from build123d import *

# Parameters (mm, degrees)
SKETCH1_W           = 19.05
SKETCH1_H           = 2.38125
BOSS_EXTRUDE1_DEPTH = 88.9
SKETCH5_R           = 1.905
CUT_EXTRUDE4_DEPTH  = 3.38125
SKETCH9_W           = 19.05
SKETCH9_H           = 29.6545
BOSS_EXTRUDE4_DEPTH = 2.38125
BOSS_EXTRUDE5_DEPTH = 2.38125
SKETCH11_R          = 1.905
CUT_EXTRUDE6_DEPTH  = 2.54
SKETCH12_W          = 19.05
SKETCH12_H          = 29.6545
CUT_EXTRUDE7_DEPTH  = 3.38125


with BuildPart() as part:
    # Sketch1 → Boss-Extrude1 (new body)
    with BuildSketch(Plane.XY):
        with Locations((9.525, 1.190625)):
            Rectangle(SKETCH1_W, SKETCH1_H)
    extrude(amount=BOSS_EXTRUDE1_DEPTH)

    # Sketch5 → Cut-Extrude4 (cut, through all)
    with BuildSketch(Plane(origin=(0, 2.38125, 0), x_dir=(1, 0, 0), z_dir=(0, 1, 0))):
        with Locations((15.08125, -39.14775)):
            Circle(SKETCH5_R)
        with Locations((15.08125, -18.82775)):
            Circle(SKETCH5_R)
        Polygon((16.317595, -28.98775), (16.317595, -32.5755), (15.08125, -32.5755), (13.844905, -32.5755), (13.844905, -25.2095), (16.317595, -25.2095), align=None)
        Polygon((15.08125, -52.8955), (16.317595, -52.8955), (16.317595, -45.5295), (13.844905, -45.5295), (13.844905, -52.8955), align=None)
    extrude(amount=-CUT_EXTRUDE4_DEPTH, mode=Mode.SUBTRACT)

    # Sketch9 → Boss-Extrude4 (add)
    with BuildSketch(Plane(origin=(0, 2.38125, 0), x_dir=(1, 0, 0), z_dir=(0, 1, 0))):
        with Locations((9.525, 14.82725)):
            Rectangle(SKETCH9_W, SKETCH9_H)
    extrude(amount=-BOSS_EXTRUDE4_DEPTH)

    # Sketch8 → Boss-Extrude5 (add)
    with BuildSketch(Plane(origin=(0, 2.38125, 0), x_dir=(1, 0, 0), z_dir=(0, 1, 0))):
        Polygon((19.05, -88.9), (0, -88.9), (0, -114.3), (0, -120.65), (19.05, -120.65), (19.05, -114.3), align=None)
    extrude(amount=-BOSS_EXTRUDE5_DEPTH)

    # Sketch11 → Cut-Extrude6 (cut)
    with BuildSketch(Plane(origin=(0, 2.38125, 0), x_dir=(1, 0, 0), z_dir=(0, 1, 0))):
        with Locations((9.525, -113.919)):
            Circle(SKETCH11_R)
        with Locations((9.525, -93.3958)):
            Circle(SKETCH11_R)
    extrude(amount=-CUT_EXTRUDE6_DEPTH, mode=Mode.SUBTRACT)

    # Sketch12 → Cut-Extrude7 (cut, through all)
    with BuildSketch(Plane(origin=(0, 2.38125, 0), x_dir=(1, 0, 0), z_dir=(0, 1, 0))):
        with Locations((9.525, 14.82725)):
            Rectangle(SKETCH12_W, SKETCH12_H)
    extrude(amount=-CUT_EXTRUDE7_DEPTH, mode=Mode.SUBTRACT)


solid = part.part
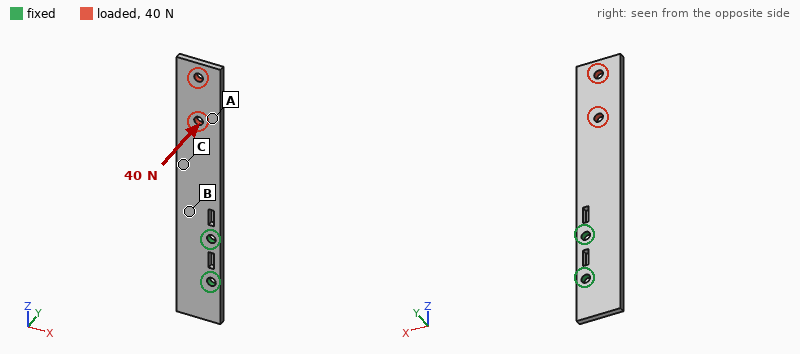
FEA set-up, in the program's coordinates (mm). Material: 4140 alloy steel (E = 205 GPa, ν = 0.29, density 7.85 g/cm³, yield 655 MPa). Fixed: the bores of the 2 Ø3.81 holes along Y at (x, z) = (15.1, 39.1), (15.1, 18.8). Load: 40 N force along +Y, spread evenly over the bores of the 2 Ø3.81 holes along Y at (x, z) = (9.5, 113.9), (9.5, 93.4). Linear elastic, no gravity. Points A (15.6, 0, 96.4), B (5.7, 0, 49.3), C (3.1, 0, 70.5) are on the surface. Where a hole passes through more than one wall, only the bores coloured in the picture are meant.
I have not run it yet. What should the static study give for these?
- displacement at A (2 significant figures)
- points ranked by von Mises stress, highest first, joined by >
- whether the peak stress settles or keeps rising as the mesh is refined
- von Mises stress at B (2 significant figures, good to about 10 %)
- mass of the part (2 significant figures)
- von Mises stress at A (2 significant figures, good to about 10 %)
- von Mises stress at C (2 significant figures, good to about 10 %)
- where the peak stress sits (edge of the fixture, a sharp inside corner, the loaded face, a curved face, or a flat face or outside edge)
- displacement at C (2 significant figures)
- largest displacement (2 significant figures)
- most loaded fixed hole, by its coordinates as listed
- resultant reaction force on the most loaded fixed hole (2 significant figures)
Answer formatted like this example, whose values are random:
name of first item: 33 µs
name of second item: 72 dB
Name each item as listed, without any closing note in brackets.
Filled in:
displacement at A: 0.73 mm
points ranked by von Mises stress, highest first, joined by >: B > C > A
whether the peak stress settles or keeps rising as the mesh is refined: keeps rising
von Mises stress at B: 130 MPa
mass of the part: 41 g
von Mises stress at A: 22 MPa
von Mises stress at C: 74 MPa
where the peak stress sits: edge of the fixture
displacement at C: 0.27 mm
largest displacement: 1.2 mm
most loaded fixed hole, by its coordinates as listed: (15.1, 39.1)
resultant reaction force on the most loaded fixed hole: 79 N
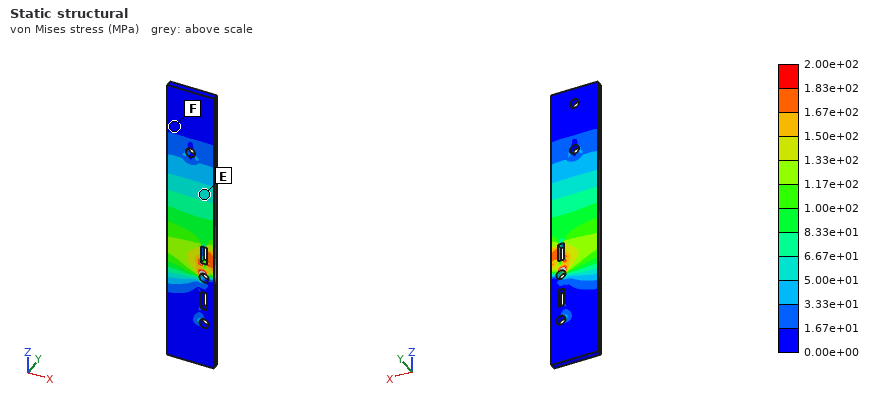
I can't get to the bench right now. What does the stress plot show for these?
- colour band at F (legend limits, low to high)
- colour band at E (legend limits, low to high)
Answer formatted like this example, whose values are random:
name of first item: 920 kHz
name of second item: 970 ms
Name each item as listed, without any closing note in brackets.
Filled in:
colour band at F: 0.00e+00 to 1.67e+01 MPa
colour band at E: 5.00e+01 to 6.67e+01 MPa
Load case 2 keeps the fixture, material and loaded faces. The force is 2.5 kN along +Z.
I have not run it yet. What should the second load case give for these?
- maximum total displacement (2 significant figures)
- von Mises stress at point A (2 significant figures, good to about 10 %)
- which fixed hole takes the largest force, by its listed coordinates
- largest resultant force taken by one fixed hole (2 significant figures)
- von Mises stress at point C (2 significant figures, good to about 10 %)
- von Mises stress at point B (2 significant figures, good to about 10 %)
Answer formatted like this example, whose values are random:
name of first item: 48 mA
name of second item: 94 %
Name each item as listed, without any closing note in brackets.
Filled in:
maximum total displacement: 36 µm
von Mises stress at point A: 42 MPa
which fixed hole takes the largest force, by its listed coordinates: (15.1, 39.1)
largest resultant force taken by one fixed hole: 1.9 kN
von Mises stress at point C: 55 MPa
von Mises stress at point B: 53 MPa
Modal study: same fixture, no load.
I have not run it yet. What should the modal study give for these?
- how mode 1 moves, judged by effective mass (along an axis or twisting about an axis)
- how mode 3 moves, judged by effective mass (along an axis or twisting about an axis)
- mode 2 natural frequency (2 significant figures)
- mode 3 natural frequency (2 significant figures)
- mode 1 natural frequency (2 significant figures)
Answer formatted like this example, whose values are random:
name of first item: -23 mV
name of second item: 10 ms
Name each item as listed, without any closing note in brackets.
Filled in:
how mode 1 moves, judged by effective mass: along Y
how mode 3 moves, judged by effective mass: along X
mode 2 natural frequency: 1800 Hz
mode 3 natural frequency: 1900 Hz
mode 1 natural frequency: 290 Hz
